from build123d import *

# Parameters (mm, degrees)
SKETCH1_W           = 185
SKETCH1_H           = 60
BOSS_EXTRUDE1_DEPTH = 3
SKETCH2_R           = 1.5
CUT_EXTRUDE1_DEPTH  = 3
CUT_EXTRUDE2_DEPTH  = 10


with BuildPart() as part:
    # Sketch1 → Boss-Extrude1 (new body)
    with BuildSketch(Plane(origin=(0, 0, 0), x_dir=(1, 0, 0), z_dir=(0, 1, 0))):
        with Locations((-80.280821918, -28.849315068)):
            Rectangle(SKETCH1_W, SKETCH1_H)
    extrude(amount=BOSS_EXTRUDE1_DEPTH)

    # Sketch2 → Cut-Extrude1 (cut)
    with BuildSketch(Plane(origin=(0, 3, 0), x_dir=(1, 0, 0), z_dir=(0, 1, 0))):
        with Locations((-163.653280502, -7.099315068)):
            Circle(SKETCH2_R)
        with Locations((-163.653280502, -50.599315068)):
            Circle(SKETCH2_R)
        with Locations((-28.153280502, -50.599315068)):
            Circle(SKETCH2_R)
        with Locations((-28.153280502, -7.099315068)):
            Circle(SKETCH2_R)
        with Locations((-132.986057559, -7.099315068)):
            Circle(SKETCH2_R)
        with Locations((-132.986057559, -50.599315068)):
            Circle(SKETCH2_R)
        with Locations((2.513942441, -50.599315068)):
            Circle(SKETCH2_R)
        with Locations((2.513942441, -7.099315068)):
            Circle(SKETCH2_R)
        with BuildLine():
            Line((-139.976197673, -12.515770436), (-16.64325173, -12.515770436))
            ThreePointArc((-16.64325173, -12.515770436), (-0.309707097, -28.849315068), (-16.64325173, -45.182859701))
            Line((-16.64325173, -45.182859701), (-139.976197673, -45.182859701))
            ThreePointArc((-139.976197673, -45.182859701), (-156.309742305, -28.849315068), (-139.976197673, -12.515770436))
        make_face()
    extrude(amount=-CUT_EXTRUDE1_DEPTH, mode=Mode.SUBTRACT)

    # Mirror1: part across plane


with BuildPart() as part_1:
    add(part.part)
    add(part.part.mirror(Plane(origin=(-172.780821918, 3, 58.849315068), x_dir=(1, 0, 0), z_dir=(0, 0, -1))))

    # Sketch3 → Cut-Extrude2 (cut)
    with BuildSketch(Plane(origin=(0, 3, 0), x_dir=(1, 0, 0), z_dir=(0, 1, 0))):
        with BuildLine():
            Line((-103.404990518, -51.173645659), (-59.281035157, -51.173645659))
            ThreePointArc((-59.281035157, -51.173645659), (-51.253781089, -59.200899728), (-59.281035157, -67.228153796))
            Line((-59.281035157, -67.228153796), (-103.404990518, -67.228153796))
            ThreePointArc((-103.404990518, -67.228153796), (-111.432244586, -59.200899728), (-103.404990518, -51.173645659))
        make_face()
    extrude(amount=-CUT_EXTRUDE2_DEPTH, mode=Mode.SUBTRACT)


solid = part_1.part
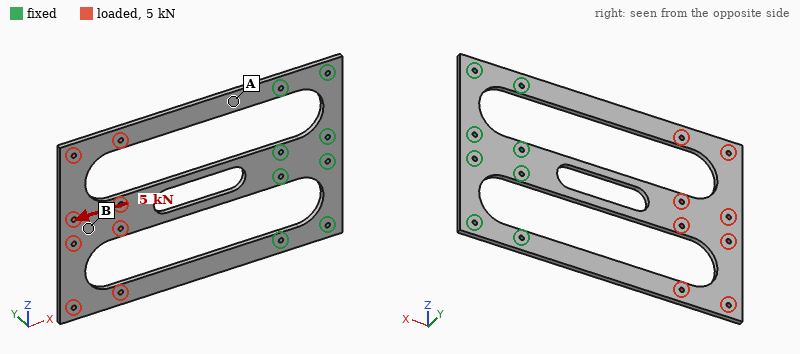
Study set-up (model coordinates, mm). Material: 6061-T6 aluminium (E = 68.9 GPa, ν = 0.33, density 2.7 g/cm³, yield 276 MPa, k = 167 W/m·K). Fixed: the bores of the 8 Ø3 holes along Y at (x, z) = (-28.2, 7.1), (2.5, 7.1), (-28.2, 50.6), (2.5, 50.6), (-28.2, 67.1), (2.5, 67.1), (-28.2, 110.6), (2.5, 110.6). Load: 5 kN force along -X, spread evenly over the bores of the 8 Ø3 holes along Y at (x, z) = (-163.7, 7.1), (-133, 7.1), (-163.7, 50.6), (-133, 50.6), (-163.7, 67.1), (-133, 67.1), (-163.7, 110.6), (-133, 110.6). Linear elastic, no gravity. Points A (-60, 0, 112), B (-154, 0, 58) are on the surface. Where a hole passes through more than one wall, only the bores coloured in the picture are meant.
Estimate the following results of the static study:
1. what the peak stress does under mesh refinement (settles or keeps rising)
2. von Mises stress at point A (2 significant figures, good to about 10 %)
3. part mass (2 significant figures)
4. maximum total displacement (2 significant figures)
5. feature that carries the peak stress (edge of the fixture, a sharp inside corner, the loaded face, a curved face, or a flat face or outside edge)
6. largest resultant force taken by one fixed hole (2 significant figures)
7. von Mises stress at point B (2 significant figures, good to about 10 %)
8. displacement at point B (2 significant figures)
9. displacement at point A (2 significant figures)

keeps rising
33 MPa
93 g
93 µm
edge of the fixture
1.2 kN
17 MPa
90 µm
25 µm
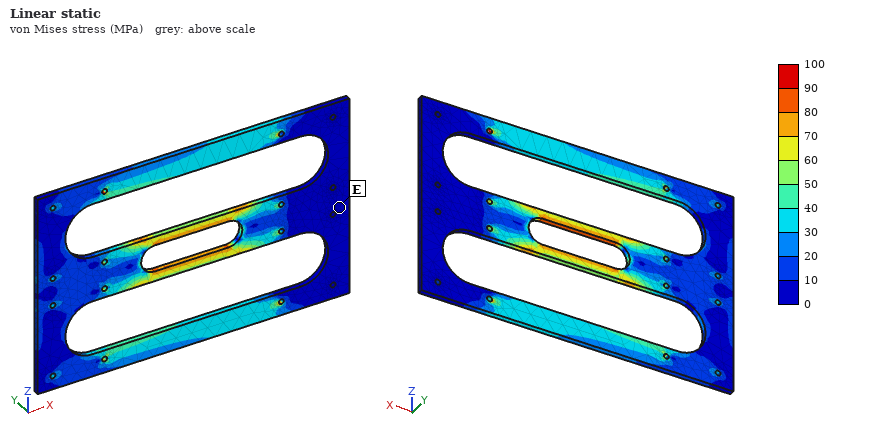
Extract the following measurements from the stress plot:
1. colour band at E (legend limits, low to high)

0 to 10 MPa
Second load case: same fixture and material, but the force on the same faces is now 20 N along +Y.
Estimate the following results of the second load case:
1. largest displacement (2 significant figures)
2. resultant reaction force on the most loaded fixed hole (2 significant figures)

2.2 mm
8.3 N
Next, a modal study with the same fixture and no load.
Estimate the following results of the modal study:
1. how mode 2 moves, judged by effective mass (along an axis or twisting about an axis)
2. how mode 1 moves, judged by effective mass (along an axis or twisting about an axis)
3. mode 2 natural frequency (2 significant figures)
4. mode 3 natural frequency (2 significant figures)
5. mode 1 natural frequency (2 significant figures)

twisting about X
along Y
240 Hz
640 Hz
86 Hz
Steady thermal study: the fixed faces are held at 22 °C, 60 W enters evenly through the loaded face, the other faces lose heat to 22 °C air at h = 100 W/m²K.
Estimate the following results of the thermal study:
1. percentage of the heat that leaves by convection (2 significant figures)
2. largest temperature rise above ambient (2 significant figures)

93 %
52 K
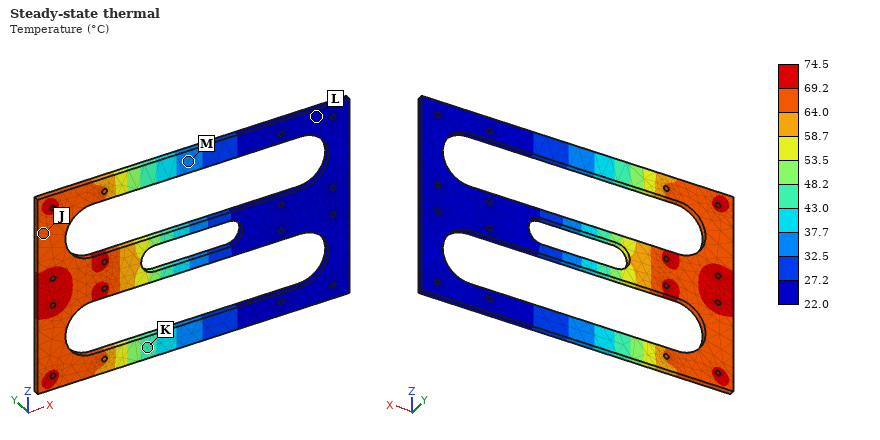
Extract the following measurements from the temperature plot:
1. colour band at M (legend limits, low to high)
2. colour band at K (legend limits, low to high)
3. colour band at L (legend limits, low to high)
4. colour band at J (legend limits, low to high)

32.5 to 37.7 °C
43.0 to 48.2 °C
22.0 to 27.2 °C
64.0 to 69.2 °C
